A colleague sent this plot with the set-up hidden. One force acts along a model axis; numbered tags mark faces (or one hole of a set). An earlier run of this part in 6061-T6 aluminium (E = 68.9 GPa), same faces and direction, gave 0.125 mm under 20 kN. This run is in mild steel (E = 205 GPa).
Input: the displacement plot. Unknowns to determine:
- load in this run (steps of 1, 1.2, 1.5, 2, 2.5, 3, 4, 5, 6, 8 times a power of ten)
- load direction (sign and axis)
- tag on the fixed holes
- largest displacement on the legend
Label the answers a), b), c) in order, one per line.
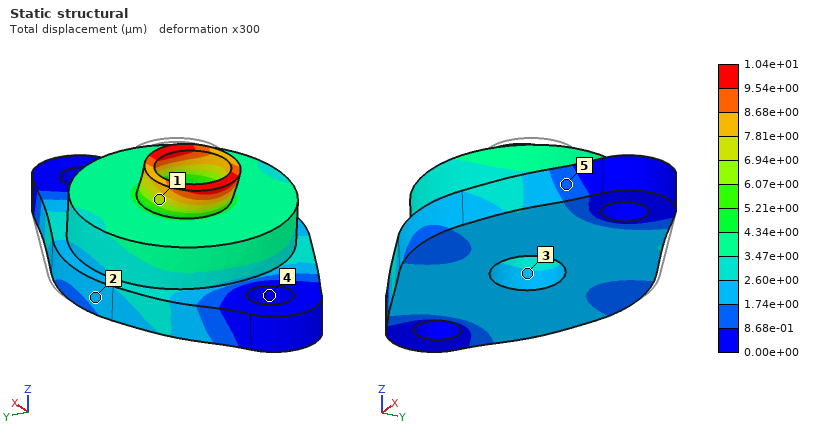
a) 5 kN
b) -X
c) 4
d) 1.04e+01 µm
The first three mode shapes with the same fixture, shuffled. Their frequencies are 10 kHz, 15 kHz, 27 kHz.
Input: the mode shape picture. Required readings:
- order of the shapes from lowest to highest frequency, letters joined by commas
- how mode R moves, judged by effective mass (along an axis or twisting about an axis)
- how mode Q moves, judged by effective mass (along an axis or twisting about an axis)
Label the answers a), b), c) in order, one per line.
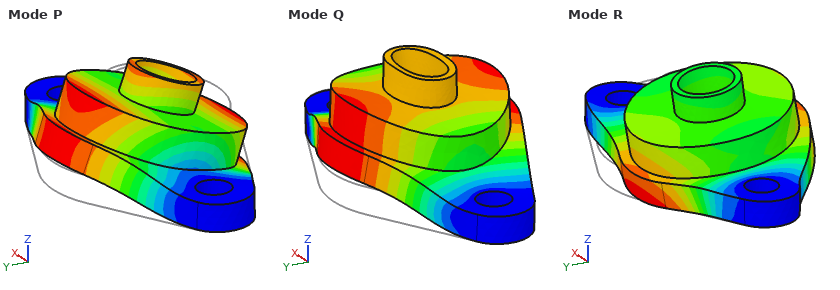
a) P, Q, R
b) along Y
c) along Z
